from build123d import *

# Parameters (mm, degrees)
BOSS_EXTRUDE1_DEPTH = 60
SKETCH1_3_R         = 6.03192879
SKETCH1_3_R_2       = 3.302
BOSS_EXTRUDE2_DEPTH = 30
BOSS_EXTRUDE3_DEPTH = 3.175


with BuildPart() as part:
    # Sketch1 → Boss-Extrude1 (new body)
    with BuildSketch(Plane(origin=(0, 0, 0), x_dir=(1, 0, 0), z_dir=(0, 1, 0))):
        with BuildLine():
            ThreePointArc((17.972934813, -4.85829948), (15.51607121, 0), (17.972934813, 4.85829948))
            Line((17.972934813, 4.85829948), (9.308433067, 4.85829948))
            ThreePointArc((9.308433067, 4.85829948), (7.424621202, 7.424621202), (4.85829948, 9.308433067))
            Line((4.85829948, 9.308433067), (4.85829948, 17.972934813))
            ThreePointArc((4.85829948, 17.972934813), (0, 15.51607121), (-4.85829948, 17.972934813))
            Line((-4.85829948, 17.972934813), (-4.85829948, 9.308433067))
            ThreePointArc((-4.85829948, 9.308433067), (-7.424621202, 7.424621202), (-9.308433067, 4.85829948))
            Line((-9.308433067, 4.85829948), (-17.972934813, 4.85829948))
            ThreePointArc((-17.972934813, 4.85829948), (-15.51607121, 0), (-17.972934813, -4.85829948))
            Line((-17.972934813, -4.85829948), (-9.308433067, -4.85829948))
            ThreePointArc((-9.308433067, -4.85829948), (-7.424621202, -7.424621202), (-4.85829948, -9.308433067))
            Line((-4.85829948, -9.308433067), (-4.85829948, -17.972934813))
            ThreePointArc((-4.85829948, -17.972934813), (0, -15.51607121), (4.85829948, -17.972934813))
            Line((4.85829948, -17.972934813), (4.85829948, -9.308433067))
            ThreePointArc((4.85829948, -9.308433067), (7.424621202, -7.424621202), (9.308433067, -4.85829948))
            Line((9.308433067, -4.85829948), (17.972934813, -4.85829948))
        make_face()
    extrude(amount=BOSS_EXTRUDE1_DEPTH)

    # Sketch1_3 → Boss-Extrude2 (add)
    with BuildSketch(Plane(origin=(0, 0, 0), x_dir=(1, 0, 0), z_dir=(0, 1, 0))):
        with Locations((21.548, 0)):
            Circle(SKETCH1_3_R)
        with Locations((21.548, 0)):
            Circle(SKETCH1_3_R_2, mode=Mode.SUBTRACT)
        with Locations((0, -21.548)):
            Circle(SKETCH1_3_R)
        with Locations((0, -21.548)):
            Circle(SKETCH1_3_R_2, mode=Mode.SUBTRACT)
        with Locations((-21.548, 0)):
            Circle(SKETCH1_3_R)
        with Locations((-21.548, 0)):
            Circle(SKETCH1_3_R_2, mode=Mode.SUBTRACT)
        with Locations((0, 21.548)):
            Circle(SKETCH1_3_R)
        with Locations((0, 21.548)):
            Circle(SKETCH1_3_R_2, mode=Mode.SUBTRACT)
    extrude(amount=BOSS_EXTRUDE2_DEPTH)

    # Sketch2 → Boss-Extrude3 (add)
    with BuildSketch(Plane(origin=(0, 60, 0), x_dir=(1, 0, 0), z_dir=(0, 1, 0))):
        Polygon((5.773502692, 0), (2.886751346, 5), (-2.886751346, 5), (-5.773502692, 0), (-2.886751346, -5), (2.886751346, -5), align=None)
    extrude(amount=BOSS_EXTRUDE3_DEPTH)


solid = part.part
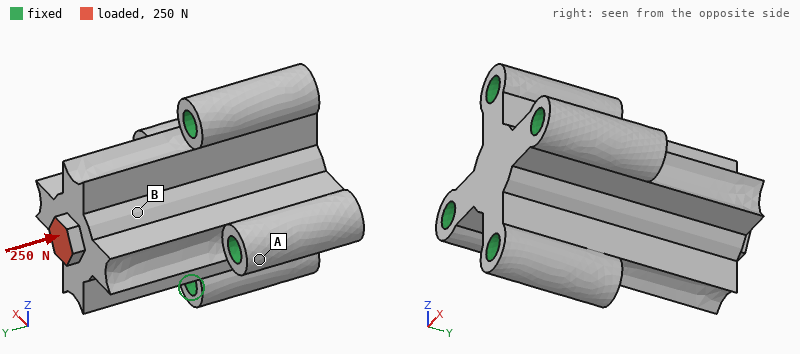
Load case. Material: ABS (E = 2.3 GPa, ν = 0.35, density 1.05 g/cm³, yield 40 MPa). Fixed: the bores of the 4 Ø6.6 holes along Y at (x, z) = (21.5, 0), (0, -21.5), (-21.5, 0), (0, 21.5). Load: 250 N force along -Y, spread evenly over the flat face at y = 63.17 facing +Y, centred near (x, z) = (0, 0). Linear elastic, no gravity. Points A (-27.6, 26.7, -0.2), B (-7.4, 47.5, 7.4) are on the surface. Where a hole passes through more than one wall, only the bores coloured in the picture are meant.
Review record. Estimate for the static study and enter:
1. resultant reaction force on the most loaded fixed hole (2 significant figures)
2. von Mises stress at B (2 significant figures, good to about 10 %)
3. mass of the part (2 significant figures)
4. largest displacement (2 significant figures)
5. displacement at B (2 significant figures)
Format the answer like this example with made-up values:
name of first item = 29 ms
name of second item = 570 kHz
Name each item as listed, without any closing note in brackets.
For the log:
resultant reaction force on the most loaded fixed hole = 69 N
von Mises stress at B = 0.50 MPa
mass of the part = 47 g
largest displacement = 17 µm
displacement at B = 6.5 µm
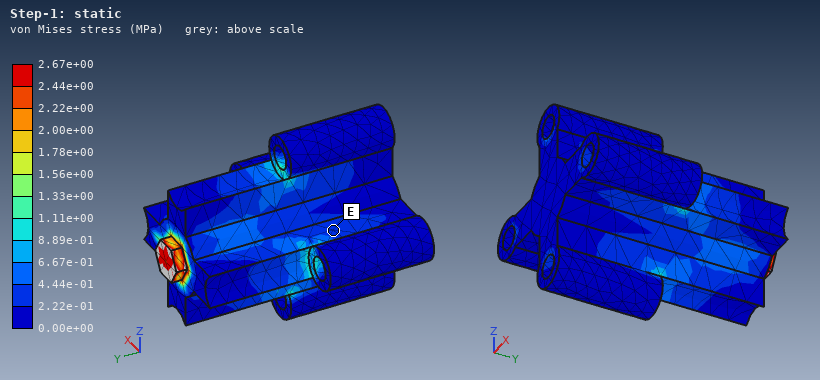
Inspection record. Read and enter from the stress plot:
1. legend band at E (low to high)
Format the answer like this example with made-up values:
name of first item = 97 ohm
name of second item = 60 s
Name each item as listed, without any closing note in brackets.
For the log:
legend band at E = 2.22e-01 to 4.44e-01 MPa
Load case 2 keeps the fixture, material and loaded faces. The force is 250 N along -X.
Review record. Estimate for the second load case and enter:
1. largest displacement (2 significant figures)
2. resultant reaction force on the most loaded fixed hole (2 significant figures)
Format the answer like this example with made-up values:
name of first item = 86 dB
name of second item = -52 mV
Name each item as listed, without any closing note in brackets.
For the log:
largest displacement = 0.12 mm
resultant reaction force on the most loaded fixed hole = 270 N
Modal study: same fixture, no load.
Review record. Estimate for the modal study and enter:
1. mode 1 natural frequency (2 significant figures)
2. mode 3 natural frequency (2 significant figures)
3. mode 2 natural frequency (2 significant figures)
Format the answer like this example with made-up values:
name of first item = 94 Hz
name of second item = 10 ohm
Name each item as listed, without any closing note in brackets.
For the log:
mode 1 natural frequency = 3400 Hz
mode 3 natural frequency = 4800 Hz
mode 2 natural frequency = 3400 Hz
